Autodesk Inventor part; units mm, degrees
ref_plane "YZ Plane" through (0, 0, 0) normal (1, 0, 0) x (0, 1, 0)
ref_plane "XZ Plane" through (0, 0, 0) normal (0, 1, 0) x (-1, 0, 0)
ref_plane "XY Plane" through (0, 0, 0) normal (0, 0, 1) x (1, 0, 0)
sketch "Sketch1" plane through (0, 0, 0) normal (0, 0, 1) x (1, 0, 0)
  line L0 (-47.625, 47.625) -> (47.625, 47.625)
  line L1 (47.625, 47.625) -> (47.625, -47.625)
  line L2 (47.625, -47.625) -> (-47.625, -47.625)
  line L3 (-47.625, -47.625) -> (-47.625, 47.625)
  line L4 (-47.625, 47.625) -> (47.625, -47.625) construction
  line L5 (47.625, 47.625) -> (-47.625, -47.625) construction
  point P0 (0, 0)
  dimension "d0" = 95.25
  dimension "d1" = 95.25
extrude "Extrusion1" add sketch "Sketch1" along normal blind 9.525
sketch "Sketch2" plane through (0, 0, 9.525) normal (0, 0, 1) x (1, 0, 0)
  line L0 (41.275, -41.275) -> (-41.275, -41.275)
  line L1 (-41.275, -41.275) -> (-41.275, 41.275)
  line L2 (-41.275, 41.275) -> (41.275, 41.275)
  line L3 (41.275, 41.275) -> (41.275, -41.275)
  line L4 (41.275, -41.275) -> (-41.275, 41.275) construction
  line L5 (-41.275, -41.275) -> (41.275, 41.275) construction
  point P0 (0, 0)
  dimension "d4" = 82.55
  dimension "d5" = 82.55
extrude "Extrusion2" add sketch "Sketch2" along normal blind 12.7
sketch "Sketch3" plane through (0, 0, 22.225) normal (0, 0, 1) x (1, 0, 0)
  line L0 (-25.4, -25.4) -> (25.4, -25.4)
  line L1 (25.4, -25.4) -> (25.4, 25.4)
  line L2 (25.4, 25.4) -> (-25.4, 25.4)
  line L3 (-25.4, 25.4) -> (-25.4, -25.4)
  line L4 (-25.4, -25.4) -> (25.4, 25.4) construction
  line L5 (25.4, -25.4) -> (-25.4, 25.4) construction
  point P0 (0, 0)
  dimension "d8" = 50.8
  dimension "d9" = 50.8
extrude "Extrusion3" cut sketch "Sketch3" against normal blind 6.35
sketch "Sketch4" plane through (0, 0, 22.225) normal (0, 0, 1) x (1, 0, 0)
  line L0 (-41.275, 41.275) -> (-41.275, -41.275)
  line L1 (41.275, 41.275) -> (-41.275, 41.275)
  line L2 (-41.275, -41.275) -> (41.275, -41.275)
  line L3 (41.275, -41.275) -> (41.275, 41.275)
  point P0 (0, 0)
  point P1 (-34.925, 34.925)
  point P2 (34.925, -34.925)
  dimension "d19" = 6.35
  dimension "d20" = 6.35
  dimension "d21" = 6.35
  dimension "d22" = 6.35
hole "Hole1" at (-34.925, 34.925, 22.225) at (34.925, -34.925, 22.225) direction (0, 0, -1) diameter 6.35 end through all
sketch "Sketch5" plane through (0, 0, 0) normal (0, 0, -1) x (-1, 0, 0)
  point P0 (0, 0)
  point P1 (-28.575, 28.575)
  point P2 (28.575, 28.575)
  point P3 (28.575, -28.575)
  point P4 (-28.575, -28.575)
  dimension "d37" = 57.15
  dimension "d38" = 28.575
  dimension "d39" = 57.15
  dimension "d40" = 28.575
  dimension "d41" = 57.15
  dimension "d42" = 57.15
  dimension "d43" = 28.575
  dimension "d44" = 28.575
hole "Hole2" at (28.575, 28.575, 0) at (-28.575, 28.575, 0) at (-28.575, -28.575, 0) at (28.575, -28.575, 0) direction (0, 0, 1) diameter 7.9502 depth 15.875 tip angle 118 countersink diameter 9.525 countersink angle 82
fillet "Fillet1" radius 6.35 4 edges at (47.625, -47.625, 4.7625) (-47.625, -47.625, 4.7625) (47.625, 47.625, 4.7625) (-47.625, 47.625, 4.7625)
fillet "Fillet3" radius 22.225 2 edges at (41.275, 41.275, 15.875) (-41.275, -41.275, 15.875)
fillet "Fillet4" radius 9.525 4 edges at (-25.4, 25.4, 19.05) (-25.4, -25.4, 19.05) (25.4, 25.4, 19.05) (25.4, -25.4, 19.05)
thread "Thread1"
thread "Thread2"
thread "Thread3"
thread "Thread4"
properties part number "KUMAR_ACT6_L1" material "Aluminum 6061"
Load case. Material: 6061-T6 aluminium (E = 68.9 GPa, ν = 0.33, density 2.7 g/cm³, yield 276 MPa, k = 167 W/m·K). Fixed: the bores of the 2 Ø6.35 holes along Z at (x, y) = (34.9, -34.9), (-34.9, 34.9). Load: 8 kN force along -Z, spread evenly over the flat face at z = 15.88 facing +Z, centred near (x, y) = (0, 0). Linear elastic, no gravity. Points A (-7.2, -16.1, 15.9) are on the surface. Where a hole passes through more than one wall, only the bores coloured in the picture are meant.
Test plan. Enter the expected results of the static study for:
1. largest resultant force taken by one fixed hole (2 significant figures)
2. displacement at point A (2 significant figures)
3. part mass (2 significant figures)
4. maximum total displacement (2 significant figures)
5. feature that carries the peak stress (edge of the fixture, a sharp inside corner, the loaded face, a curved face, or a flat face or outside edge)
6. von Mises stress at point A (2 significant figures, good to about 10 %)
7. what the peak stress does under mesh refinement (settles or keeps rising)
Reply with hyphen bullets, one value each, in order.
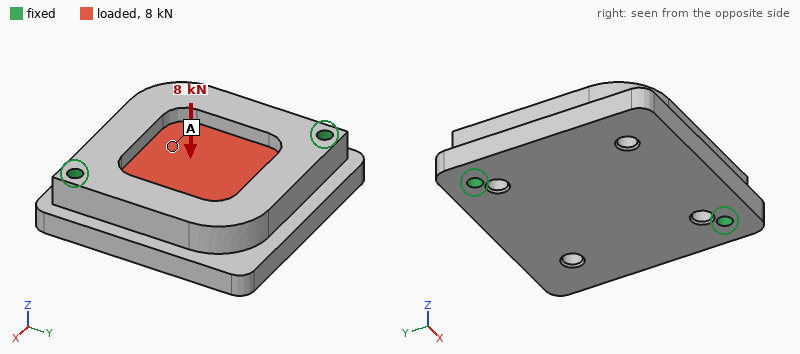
- 4.2 kN
- 28 µm
- 400 g
- 36 µm
- edge of the fixture
- 12 MPa
- keeps rising
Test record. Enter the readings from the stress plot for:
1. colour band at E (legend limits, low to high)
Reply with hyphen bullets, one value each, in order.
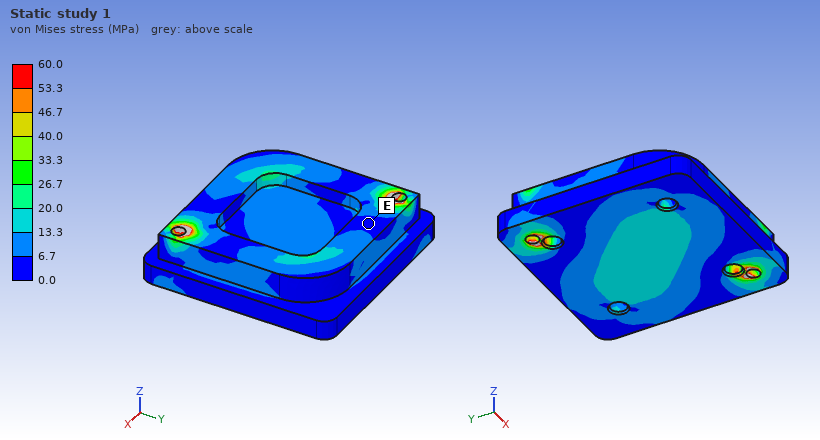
- 0.0 to 6.7 MPa
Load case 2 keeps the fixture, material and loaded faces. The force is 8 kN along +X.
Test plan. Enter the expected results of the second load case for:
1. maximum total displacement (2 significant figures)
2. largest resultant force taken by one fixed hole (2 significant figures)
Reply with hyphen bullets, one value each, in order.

- 15 µm
- 4.0 kN
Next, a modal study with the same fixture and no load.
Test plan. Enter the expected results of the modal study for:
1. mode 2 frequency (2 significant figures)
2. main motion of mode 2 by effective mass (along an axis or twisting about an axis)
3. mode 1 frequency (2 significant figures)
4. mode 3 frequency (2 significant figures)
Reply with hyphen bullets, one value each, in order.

- 4400 Hz
- along Z
- 3500 Hz
- 9600 Hz
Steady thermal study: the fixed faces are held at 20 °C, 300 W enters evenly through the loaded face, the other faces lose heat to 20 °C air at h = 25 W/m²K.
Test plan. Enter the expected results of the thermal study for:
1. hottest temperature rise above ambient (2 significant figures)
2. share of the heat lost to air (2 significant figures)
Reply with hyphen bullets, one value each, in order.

- 47 K
- 5.9 %
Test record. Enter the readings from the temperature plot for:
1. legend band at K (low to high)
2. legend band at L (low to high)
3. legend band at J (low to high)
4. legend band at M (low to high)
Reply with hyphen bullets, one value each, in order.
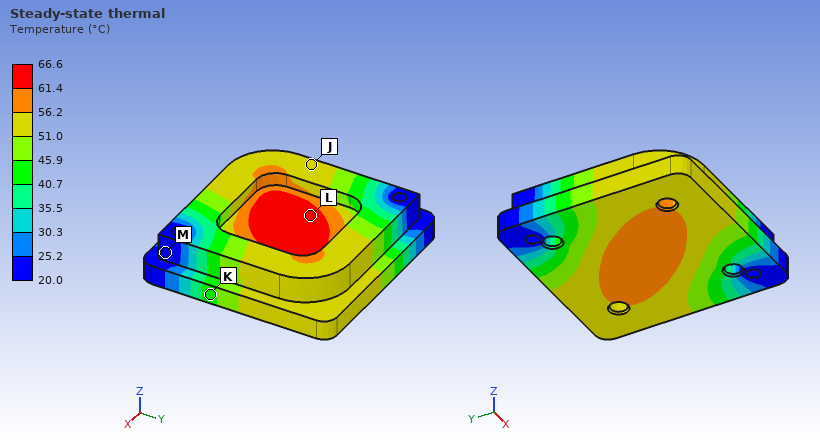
- 40.7 to 45.9 °C
- 61.4 to 66.6 °C
- 51.0 to 56.2 °C
- 20.0 to 25.2 °C
